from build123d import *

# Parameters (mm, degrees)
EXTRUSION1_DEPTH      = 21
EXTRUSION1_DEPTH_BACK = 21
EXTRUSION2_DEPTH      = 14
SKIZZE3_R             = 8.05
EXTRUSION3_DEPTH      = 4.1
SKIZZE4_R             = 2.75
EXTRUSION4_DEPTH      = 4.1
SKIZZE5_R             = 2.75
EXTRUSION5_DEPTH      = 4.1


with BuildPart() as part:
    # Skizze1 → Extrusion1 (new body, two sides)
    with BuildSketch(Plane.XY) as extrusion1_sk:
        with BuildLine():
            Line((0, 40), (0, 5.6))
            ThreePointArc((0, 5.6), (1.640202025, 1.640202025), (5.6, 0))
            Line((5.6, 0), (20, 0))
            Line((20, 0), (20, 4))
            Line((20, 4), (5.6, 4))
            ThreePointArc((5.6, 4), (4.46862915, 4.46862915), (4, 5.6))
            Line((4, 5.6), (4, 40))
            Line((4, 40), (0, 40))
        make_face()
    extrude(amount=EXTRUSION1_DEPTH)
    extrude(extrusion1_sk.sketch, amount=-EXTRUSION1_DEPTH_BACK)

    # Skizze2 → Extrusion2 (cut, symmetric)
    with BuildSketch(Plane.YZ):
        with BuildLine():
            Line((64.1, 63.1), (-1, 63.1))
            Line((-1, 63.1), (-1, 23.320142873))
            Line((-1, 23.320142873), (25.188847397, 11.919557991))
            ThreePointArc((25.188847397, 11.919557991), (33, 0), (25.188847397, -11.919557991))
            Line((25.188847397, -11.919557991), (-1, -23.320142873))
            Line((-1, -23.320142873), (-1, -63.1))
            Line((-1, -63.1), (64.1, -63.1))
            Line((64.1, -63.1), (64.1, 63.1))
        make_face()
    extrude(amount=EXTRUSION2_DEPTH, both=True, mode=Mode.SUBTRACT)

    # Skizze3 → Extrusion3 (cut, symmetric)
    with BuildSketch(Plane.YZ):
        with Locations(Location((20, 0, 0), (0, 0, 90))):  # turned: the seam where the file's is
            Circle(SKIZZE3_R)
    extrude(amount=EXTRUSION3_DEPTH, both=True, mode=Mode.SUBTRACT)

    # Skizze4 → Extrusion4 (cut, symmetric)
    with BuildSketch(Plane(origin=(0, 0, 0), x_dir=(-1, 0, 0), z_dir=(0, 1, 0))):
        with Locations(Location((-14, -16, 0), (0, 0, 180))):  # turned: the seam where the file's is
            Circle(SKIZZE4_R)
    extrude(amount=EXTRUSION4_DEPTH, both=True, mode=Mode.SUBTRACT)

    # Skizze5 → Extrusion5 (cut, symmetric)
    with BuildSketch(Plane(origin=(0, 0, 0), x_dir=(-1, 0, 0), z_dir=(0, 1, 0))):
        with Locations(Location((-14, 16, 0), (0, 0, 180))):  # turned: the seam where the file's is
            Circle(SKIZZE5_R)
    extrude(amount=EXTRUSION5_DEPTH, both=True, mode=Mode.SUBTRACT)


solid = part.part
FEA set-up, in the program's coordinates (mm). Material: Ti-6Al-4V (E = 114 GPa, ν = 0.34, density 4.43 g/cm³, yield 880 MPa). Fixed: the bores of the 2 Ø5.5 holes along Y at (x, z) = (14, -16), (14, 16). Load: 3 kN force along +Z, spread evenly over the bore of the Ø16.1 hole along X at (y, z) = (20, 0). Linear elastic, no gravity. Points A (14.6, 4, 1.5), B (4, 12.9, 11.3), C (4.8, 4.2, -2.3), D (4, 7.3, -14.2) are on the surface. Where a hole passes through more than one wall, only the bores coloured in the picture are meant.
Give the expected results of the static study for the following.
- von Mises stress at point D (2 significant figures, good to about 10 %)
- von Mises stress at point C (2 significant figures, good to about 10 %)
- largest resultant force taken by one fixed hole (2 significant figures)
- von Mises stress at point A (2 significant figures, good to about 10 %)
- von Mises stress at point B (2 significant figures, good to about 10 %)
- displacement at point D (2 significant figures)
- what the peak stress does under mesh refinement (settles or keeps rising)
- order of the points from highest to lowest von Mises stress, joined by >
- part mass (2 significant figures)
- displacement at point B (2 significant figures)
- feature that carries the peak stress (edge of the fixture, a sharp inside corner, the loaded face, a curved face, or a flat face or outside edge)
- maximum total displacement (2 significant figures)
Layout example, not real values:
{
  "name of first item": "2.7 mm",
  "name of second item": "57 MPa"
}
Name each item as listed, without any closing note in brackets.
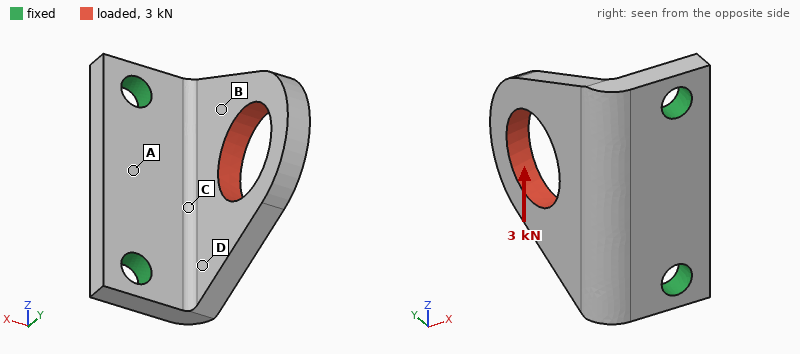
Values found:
{
  "von Mises stress at point D": "120 MPa",
  "von Mises stress at point C": "190 MPa",
  "largest resultant force taken by one fixed hole": "2.4 kN",
  "von Mises stress at point A": "40 MPa",
  "von Mises stress at point B": "64 MPa",
  "displacement at point D": "0.047 mm",
  "what the peak stress does under mesh refinement": "keeps rising",
  "order of the points from highest to lowest von Mises stress, joined by >": "C > D > B > A",
  "part mass": "24 g",
  "displacement at point B": "0.062 mm",
  "feature that carries the peak stress": "edge of the fixture",
  "maximum total displacement": "0.14 mm"
}
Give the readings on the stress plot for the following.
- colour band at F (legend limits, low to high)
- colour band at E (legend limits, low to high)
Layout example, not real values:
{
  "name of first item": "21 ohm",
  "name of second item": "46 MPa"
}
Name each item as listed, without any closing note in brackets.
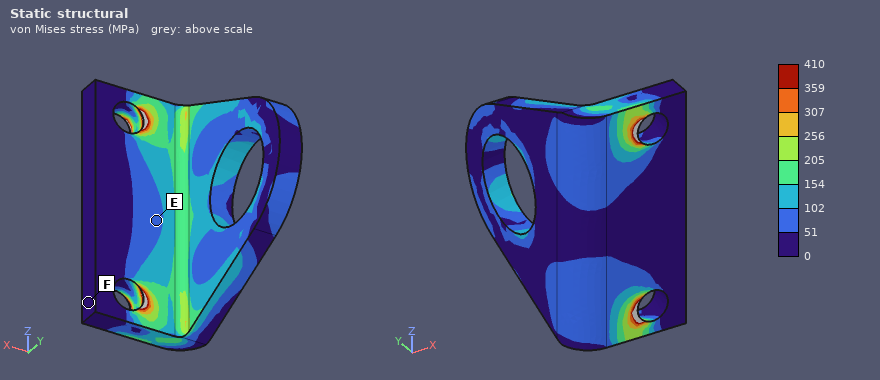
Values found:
{
  "colour band at F": "0 to 51 MPa",
  "colour band at E": "51 to 102 MPa"
}
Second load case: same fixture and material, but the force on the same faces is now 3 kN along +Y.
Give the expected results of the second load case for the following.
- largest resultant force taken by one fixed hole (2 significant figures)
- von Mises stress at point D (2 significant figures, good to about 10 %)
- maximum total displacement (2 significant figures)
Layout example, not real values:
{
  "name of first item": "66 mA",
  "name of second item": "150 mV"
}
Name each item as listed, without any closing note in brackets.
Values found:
{
  "largest resultant force taken by one fixed hole": "1.5 kN",
  "von Mises stress at point D": "46 MPa",
  "maximum total displacement": "0.27 mm"
}
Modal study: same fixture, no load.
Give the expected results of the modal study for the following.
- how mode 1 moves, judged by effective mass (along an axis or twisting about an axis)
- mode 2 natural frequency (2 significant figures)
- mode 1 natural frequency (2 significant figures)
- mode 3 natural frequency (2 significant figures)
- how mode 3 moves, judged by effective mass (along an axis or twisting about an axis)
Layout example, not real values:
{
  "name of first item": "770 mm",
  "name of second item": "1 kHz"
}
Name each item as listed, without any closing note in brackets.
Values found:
{
  "how mode 1 moves, judged by effective mass": "along X",
  "mode 2 natural frequency": "8200 Hz",
  "mode 1 natural frequency": "3500 Hz",
  "mode 3 natural frequency": "10 kHz",
  "how mode 3 moves, judged by effective mass": "along Y"
}
